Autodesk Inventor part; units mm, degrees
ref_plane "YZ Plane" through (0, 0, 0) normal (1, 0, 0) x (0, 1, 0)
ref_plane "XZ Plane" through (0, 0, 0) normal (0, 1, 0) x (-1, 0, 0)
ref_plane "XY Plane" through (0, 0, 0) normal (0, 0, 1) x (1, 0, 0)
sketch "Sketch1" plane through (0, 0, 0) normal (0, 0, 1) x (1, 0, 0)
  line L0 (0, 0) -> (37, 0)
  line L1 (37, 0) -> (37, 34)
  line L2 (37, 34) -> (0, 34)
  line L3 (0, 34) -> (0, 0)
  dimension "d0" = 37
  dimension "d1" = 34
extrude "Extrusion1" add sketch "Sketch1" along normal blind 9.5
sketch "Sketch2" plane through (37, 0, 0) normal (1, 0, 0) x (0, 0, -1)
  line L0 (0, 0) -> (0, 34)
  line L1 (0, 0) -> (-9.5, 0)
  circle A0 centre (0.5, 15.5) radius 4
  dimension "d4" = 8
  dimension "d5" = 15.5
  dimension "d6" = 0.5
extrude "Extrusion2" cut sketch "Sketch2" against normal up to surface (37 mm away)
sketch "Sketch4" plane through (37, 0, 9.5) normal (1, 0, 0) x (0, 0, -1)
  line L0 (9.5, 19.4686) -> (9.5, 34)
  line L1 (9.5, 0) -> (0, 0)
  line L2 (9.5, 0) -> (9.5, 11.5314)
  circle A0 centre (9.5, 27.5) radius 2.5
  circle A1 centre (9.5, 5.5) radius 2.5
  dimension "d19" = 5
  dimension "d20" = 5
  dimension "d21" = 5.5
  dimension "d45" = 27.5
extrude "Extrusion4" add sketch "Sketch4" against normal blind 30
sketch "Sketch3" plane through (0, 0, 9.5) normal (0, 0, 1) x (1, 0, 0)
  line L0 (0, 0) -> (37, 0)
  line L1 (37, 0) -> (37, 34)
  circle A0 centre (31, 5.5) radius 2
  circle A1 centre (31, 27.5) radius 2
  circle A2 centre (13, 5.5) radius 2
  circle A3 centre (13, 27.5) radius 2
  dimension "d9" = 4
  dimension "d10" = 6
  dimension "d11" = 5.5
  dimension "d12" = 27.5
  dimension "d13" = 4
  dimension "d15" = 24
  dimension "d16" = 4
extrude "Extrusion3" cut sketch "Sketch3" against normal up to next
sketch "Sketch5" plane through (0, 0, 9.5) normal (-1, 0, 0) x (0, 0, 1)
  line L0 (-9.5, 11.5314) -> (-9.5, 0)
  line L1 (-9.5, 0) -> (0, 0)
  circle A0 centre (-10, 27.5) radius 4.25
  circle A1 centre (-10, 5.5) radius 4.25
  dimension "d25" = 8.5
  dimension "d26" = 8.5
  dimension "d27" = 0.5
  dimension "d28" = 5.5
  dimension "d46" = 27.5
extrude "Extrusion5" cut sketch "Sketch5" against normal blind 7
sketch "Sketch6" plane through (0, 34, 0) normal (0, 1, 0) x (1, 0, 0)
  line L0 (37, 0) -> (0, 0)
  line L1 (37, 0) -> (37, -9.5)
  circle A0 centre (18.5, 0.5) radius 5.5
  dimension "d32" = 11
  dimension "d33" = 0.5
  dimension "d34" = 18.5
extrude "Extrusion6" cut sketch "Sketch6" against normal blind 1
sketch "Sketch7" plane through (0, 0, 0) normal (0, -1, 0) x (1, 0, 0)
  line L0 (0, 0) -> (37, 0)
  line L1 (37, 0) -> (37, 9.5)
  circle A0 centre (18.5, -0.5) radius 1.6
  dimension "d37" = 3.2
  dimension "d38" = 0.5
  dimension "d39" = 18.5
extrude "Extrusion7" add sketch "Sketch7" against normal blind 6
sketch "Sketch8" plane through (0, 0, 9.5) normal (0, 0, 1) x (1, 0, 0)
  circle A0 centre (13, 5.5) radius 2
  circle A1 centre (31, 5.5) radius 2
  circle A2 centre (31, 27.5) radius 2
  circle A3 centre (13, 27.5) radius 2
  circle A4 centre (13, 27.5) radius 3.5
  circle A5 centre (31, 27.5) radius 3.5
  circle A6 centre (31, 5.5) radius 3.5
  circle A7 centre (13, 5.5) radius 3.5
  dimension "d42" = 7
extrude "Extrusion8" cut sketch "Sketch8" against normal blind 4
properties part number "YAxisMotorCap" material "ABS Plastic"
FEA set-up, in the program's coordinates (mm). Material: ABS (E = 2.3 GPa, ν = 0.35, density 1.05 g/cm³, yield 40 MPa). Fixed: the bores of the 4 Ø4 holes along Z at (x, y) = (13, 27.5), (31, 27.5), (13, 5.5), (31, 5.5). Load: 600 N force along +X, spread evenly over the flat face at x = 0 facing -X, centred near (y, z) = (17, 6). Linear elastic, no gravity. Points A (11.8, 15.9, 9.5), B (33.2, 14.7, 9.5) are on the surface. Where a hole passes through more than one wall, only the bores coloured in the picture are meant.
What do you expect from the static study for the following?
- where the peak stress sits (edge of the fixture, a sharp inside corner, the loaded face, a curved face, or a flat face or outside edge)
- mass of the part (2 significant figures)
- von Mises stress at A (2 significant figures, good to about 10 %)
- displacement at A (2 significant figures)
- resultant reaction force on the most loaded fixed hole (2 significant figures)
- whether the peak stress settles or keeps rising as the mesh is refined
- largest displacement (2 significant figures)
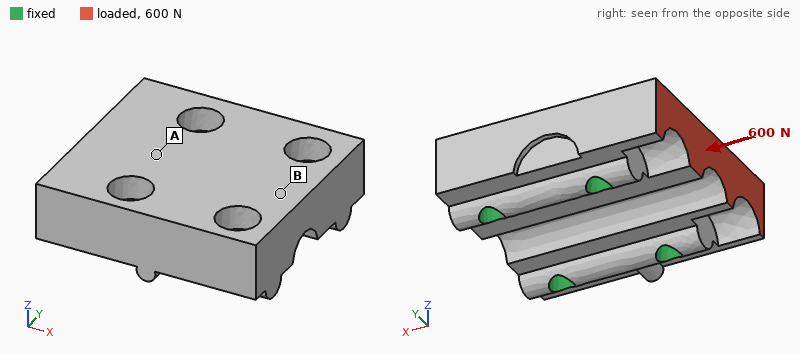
edge of the fixture
11 g
2.6 MPa
18 µm
240 N
keeps rising
42 µm
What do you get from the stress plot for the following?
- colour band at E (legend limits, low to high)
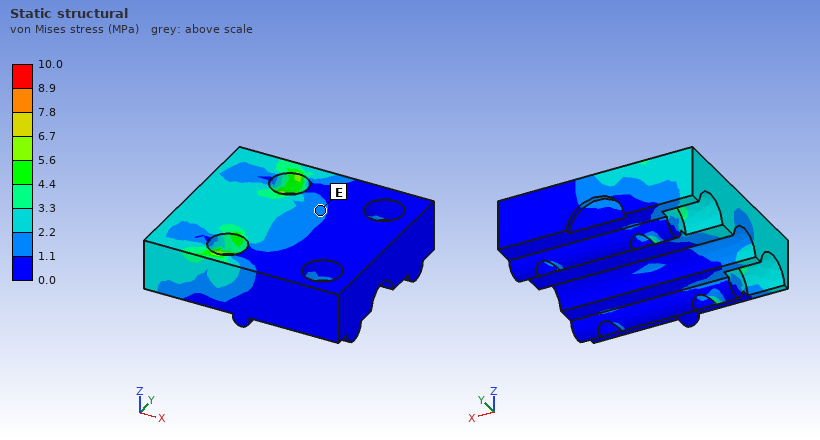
1.1 to 2.2 MPa
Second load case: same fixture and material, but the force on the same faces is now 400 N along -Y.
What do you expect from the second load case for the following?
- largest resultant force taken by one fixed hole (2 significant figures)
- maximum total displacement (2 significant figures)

270 N
77 µm
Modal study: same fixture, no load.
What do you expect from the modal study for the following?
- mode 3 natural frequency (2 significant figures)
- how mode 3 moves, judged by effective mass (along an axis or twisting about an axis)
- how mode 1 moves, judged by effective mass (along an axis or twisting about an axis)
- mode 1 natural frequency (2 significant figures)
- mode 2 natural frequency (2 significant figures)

13 kHz
along Y
along Z
7700 Hz
10 kHz
